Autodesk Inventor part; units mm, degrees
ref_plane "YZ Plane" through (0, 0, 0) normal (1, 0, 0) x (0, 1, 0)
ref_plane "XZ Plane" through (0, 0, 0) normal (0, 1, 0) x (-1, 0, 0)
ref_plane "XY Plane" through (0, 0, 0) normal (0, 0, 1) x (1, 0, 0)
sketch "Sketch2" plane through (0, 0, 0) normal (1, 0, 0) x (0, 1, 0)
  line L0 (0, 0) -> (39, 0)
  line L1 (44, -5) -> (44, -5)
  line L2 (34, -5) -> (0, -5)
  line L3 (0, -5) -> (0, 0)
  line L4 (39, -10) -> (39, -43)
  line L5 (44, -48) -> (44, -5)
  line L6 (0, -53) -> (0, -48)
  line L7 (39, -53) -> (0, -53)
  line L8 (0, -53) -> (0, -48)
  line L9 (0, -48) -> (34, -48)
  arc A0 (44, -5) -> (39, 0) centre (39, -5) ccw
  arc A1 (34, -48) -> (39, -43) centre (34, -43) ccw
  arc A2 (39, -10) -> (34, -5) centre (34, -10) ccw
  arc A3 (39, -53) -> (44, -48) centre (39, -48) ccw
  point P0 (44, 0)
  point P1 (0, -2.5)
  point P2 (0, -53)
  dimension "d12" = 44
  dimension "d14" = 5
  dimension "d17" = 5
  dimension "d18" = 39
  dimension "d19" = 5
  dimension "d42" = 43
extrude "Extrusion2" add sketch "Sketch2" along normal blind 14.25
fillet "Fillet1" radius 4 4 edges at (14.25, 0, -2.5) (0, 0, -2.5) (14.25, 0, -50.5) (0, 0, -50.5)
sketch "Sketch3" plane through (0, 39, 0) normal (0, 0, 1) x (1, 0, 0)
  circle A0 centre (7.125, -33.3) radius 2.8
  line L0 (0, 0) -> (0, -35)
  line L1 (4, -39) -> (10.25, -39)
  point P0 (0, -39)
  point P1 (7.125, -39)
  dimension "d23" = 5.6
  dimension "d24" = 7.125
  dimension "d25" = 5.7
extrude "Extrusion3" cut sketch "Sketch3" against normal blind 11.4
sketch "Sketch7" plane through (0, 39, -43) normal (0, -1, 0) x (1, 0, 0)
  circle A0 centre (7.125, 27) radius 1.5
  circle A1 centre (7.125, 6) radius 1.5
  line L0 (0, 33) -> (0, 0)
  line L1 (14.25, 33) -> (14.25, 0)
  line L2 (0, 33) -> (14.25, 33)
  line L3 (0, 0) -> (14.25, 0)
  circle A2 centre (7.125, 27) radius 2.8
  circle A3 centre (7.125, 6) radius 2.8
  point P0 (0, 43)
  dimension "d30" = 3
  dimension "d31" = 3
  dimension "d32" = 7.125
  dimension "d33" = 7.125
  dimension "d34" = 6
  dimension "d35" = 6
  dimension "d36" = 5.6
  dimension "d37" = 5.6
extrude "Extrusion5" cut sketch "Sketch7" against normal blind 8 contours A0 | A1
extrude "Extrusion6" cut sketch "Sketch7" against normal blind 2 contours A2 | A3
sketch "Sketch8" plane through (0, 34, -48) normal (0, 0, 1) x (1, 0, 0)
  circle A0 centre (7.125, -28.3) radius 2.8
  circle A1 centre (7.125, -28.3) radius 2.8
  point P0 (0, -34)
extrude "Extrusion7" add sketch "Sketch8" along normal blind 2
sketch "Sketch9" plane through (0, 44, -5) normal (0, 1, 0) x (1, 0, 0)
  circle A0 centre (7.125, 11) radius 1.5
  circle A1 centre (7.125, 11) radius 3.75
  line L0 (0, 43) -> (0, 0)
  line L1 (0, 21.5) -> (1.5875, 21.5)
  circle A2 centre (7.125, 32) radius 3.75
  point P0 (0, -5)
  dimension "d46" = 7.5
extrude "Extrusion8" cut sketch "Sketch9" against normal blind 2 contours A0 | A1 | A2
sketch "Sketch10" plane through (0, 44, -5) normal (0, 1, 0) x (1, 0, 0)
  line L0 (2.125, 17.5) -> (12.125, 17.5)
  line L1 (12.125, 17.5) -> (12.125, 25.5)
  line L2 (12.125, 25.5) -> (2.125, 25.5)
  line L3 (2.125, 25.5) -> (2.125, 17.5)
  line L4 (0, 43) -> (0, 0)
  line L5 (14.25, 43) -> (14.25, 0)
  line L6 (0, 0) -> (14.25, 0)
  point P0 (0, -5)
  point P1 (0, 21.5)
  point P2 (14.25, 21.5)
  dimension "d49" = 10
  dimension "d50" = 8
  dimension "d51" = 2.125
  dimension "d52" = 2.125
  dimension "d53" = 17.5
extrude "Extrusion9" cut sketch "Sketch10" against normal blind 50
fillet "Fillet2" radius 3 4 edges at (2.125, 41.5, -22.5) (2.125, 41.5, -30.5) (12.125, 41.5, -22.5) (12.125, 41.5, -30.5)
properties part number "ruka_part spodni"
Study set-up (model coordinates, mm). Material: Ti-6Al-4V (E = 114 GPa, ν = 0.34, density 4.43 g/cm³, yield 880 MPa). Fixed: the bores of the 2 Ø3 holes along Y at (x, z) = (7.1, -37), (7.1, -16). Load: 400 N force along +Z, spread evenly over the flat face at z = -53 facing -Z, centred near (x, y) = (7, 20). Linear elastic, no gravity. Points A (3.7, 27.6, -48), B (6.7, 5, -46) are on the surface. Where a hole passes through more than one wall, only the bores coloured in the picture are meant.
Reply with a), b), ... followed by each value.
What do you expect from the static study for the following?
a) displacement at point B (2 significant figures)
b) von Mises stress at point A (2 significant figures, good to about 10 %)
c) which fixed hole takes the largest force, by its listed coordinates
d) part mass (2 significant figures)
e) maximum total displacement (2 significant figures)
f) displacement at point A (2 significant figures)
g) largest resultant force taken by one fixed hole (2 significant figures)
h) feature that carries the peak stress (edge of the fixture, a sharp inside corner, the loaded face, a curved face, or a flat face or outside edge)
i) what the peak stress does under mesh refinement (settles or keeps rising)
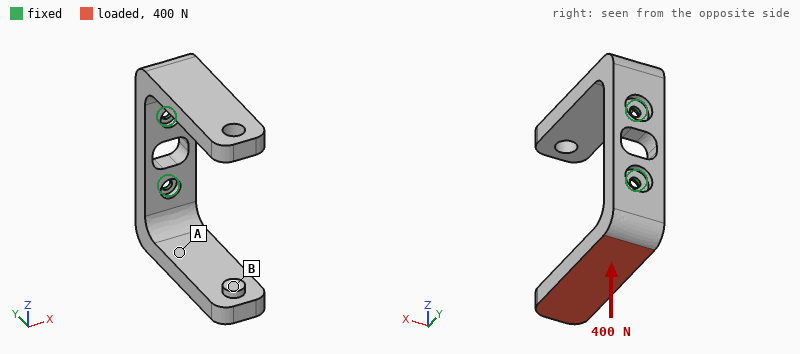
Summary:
a) 0.59 mm
b) 64 MPa
c) (7.1, -37)
d) 38 g
e) 0.71 mm
f) 0.22 mm
g) 450 N
h) edge of the fixture
i) keeps rising
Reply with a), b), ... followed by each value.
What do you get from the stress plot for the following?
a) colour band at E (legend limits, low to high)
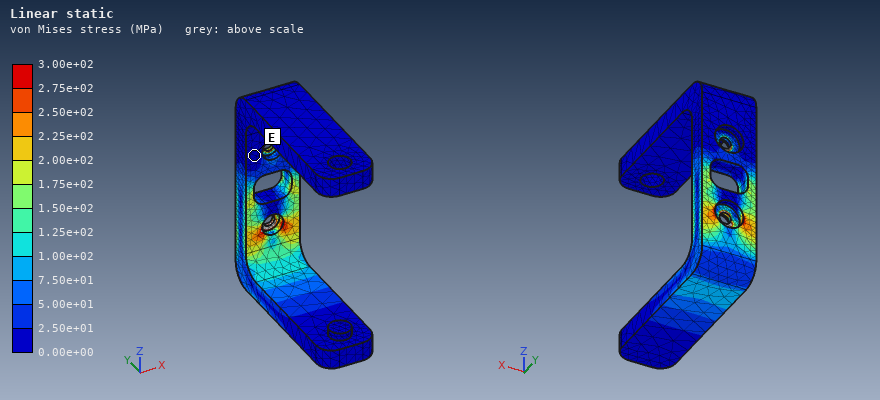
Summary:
a) 0.00e+00 to 2.50e+01 MPa
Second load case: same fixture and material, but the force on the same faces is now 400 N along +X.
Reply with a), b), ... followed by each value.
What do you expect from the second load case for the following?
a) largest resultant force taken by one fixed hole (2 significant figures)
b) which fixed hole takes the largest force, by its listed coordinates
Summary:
a) 600 N
b) (7.1, -37)
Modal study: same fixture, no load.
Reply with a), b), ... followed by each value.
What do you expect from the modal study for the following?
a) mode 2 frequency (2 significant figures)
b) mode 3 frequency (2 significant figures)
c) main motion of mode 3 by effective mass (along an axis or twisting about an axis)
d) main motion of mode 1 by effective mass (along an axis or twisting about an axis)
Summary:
a) 1200 Hz
b) 1400 Hz
c) along Z
d) along X
